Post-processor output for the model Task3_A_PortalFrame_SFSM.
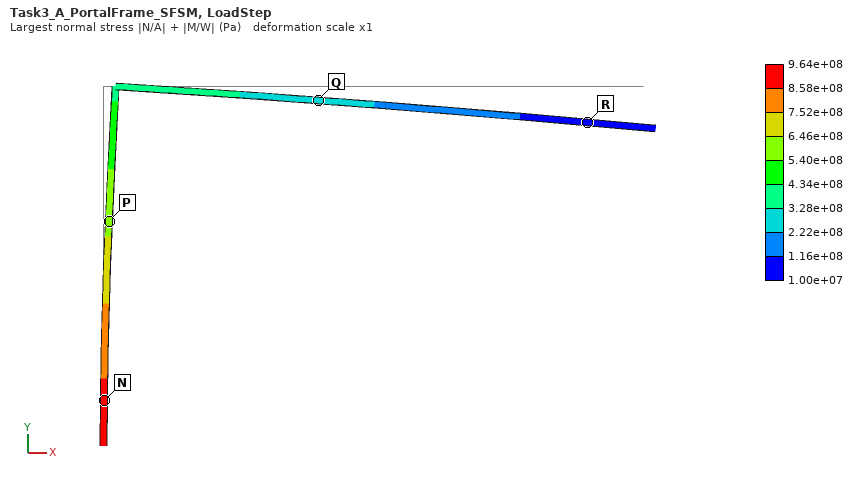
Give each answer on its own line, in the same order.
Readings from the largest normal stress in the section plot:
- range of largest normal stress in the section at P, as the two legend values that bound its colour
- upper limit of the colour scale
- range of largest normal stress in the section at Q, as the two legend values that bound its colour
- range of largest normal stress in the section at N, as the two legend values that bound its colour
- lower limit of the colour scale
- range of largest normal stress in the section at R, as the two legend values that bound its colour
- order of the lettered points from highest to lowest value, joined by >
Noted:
5.40e+08 to 6.46e+08 Pa
9.64e+08 Pa
2.22e+08 to 3.28e+08 Pa
8.58e+08 to 9.64e+08 Pa
1.00e+07 Pa
1.00e+07 to 1.16e+08 Pa
N > P > Q > R
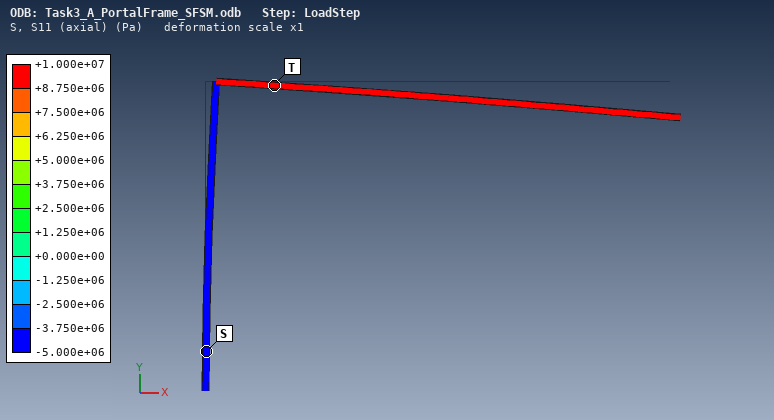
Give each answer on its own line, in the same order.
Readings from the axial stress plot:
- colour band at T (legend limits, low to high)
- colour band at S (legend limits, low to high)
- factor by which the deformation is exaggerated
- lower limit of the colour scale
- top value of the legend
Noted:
+8.750e+06 to +1.000e+07 Pa
-5.000e+06 to -3.750e+06 Pa
1
-5.000e+06 Pa
+1.000e+07 Pa
